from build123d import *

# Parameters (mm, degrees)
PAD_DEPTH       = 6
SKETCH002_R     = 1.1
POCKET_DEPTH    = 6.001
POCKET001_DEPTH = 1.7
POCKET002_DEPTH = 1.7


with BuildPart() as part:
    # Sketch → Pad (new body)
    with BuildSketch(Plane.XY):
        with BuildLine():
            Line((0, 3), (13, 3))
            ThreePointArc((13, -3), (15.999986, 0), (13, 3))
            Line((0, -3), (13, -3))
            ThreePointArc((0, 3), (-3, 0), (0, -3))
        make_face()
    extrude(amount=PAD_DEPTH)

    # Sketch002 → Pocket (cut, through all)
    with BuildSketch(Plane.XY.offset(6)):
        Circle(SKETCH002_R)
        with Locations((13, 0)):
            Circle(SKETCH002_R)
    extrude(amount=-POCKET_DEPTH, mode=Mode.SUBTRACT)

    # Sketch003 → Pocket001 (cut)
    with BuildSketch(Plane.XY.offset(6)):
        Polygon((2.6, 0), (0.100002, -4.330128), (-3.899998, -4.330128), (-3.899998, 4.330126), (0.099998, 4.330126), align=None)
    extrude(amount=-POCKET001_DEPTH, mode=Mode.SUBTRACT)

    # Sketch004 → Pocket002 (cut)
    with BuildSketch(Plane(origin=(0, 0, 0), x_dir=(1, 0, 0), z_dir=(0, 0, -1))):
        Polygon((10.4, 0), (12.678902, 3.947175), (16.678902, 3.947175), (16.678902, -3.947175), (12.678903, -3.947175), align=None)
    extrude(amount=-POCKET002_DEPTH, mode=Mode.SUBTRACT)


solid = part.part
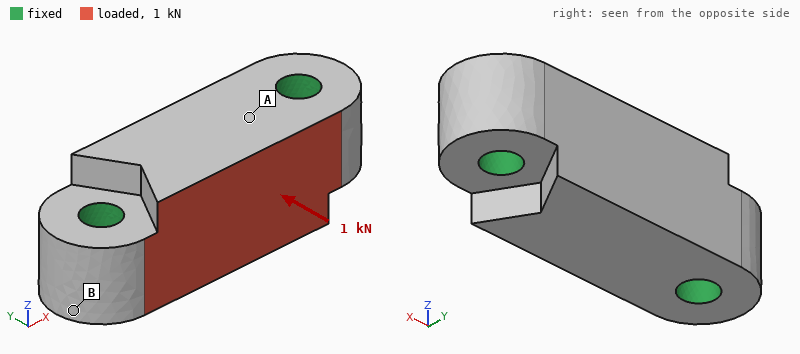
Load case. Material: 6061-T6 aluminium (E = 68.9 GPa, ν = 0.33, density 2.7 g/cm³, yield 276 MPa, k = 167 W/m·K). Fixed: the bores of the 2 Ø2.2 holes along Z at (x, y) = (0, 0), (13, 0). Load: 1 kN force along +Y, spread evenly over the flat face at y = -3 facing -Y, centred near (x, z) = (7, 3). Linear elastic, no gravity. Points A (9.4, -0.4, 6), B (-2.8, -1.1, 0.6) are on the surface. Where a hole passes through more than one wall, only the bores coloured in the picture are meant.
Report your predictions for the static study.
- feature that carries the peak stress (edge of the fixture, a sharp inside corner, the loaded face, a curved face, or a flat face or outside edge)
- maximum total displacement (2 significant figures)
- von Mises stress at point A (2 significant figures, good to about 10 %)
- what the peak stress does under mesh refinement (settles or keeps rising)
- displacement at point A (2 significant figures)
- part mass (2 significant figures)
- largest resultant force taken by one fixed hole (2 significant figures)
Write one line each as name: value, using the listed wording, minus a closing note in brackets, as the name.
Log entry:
feature that carries the peak stress: edge of the fixture
maximum total displacement: 4.5 µm
von Mises stress at point A: 22 MPa
what the peak stress does under mesh refinement: keeps rising
displacement at point A: 2.7 µm
part mass: 1.4 g
largest resultant force taken by one fixed hole: 500 N
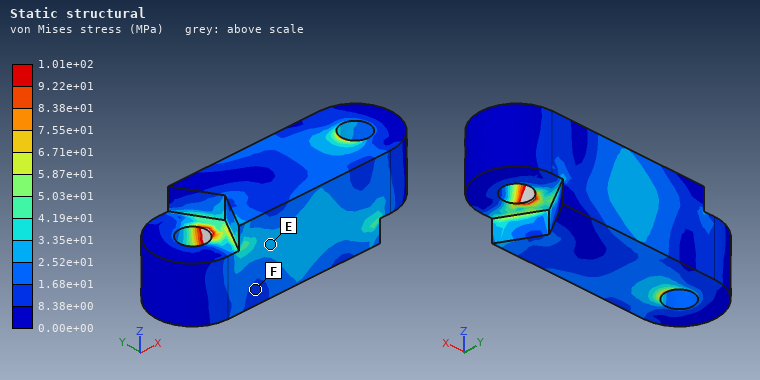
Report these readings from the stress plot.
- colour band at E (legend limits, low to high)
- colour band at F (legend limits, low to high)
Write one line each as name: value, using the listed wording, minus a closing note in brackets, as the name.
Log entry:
colour band at E: 2.52e+01 to 3.35e+01 MPa
colour band at F: 8.38e+00 to 1.68e+01 MPa
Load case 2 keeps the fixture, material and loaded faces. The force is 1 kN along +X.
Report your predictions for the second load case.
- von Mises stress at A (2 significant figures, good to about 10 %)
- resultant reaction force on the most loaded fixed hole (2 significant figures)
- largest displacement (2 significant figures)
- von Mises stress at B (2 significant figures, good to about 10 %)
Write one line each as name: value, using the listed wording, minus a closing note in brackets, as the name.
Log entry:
von Mises stress at A: 16 MPa
resultant reaction force on the most loaded fixed hole: 540 N
largest displacement: 5.3 µm
von Mises stress at B: 6.8 MPa
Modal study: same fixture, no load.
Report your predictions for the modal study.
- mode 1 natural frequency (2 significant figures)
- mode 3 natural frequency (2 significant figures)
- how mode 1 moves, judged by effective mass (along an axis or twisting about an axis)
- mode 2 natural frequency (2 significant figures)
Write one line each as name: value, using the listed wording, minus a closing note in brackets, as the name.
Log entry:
mode 1 natural frequency: 81 kHz
mode 3 natural frequency: 87 kHz
how mode 1 moves, judged by effective mass: along Y
mode 2 natural frequency: 87 kHz
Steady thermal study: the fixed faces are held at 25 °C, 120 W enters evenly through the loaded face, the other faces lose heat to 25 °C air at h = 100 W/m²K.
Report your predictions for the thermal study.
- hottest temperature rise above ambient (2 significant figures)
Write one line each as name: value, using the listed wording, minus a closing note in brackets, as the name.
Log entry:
hottest temperature rise above ambient: 59 K
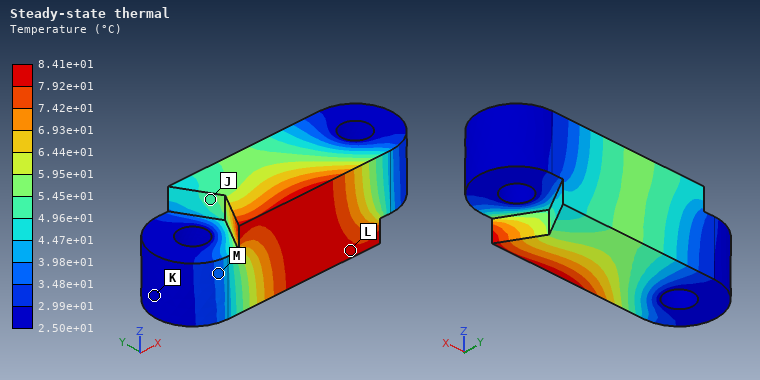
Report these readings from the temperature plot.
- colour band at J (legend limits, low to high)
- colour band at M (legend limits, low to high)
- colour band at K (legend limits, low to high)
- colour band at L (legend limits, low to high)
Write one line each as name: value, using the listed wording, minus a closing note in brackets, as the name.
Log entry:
colour band at J: 4.96e+01 to 5.45e+01 °C
colour band at M: 3.48e+01 to 3.98e+01 °C
colour band at K: 2.50e+01 to 2.99e+01 °C
colour band at L: 7.92e+01 to 8.41e+01 °C
